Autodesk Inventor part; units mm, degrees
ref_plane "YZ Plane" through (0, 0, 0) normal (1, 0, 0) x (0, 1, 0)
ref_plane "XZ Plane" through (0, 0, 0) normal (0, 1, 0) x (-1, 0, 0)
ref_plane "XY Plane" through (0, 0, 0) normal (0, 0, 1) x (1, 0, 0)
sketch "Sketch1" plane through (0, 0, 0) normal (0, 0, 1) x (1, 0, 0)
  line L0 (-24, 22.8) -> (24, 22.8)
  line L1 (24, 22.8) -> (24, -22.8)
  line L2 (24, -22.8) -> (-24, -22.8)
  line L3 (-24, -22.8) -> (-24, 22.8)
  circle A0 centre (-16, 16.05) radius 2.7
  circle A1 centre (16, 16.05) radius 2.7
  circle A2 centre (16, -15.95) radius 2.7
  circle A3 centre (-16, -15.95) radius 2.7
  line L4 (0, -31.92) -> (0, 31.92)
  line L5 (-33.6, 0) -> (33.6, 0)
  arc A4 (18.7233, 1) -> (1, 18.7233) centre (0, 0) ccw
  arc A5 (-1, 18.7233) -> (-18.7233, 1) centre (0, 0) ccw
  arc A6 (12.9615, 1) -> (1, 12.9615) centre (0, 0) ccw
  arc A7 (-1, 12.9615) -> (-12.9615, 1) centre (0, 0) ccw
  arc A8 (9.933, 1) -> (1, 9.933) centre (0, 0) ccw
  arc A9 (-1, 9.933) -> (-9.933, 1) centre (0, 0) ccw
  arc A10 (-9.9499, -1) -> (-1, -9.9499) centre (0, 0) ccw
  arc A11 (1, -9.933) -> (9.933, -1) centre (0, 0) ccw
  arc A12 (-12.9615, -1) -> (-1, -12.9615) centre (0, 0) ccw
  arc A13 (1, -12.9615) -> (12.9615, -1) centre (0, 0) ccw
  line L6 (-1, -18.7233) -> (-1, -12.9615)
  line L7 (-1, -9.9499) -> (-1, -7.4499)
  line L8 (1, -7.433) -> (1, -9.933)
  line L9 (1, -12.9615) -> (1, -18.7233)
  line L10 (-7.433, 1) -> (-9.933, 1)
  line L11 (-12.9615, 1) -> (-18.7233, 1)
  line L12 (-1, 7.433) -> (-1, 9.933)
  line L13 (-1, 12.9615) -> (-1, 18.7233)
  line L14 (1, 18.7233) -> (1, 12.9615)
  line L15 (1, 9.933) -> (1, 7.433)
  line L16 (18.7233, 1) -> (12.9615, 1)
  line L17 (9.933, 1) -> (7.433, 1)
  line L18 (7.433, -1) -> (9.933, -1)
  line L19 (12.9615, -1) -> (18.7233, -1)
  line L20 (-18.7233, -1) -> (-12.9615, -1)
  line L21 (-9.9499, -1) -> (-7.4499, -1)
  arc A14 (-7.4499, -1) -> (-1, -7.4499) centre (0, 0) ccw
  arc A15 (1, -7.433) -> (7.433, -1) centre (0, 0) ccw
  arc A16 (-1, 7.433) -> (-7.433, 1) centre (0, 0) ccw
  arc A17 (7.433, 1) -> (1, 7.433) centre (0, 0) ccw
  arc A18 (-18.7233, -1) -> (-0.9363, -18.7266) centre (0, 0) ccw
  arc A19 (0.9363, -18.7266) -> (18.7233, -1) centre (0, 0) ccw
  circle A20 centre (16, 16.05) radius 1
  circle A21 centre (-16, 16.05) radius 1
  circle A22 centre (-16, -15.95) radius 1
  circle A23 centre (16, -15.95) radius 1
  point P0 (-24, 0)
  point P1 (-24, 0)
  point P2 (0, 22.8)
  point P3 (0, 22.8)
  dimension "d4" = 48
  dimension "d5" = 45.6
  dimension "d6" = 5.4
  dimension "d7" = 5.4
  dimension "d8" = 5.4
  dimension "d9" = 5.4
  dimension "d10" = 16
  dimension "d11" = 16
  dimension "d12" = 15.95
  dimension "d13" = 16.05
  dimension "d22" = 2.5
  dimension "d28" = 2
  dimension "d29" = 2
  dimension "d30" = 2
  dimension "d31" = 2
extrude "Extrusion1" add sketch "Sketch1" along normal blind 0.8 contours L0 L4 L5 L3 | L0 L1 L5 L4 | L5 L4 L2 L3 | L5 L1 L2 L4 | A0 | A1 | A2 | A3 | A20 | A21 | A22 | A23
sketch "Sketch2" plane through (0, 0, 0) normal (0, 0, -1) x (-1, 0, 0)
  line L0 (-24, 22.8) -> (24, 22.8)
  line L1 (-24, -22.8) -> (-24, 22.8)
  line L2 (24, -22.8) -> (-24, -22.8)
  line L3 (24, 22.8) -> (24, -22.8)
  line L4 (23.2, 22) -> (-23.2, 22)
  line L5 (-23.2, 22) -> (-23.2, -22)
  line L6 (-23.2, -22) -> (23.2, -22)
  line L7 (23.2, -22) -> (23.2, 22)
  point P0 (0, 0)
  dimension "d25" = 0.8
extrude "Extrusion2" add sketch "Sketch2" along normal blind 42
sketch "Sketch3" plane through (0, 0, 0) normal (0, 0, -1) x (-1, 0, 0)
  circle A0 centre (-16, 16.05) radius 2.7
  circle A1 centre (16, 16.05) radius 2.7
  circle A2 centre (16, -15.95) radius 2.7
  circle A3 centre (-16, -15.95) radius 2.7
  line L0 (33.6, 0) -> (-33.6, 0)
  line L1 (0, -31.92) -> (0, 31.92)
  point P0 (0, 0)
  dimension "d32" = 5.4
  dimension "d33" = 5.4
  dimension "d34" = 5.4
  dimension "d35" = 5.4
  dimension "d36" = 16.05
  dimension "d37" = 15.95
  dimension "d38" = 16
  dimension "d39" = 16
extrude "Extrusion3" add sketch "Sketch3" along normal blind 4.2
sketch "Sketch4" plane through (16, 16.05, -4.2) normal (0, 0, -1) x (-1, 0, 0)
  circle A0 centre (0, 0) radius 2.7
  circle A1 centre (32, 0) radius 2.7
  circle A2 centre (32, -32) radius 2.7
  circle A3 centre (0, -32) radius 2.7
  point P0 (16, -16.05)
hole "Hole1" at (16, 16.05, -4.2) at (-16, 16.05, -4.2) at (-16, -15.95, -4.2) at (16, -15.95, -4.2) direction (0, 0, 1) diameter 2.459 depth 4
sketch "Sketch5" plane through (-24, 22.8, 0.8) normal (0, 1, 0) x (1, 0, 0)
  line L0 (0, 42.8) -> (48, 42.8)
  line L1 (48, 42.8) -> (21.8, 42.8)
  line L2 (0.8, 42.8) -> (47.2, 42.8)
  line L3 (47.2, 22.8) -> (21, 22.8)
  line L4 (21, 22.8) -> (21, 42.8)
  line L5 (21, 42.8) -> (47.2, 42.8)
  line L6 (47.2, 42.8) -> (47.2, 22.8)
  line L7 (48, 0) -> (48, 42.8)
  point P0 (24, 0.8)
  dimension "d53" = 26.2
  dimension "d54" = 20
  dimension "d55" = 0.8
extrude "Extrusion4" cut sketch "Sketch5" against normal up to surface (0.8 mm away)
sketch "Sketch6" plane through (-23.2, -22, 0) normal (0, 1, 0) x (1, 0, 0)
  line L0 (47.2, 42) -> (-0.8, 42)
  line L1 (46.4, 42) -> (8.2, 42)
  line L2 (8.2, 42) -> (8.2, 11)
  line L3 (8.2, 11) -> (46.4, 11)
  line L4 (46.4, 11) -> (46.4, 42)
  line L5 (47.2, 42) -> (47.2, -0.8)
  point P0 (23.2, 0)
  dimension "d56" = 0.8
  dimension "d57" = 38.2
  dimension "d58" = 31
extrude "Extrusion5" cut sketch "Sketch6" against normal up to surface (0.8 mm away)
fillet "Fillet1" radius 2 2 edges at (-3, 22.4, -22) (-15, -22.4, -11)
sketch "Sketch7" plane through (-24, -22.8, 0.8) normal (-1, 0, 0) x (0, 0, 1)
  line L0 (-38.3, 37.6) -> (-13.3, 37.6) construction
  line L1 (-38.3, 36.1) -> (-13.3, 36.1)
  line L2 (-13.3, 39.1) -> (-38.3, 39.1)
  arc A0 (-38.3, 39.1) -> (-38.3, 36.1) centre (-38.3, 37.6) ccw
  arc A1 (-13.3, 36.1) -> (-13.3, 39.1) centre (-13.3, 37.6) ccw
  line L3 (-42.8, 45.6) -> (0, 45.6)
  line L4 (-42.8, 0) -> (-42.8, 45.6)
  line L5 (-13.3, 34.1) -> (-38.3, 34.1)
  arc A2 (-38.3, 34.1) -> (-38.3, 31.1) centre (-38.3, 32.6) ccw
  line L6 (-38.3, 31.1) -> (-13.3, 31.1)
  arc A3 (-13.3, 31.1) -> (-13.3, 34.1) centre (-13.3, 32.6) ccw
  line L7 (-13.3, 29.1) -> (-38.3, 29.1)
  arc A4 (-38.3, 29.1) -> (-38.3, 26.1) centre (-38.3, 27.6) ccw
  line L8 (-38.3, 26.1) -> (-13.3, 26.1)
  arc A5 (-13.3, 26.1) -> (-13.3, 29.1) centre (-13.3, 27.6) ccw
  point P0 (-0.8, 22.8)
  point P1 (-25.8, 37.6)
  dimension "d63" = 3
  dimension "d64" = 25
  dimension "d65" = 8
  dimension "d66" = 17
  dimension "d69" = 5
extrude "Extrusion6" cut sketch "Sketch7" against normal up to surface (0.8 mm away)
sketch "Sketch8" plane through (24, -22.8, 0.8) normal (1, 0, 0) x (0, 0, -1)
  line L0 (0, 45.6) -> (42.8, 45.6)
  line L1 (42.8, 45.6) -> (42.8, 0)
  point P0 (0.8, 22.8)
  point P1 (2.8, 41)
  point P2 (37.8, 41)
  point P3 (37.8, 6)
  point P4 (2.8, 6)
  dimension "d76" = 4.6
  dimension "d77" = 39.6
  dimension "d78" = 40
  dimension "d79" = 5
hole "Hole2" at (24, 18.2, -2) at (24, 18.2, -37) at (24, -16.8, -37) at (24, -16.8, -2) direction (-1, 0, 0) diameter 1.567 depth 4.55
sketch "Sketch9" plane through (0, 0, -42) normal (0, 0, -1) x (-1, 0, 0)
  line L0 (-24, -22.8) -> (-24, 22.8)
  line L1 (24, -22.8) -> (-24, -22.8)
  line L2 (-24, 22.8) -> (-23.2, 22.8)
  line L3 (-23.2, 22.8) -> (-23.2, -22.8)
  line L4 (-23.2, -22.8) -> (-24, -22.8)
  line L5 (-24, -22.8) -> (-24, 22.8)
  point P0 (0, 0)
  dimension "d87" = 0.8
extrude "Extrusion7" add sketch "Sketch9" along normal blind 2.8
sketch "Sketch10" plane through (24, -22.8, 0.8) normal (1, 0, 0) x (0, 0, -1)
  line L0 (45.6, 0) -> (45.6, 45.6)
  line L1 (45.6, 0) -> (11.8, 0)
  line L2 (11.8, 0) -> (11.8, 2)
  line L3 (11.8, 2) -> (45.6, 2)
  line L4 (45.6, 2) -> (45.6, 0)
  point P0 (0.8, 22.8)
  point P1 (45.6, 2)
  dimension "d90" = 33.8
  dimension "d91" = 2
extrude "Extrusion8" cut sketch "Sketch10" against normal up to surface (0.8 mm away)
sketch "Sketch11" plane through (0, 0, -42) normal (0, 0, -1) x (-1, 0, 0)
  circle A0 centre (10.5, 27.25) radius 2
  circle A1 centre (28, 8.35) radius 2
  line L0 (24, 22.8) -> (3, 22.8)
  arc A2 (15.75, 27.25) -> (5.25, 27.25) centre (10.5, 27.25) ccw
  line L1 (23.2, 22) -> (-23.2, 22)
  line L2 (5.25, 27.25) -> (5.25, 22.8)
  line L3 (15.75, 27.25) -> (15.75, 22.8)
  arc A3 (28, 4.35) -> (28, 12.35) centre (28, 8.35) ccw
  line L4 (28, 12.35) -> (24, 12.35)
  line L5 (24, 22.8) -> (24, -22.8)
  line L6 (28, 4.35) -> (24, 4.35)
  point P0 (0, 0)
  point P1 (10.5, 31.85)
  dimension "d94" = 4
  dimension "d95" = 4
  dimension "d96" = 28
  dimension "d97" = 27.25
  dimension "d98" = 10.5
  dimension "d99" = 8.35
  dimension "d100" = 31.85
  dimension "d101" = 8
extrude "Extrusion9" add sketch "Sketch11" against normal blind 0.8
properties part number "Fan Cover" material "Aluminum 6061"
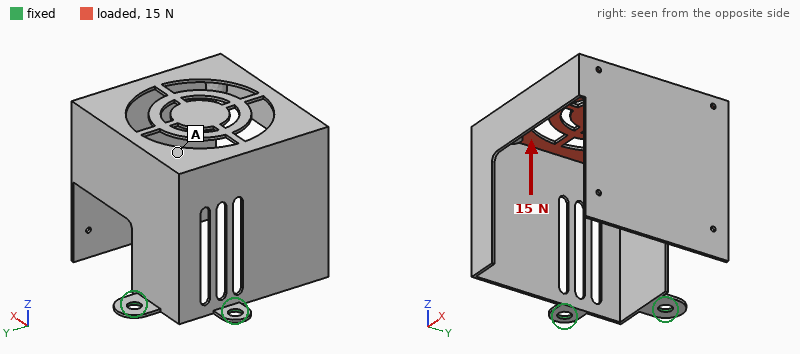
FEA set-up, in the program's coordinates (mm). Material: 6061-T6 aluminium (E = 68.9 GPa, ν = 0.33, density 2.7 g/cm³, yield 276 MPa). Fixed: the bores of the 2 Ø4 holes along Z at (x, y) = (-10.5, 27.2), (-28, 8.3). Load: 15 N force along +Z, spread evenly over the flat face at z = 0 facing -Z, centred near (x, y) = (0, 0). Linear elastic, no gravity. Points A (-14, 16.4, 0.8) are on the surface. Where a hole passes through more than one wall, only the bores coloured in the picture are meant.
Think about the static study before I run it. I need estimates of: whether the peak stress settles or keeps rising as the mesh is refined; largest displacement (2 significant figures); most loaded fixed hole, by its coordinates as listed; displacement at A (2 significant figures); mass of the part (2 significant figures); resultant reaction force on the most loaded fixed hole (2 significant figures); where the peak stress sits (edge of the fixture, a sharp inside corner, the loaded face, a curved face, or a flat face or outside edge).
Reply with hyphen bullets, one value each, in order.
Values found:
- keeps rising
- 1.0 mm
- (-28, 8.3)
- 0.44 mm
- 17 g
- 9.4 N
- edge of the fixture
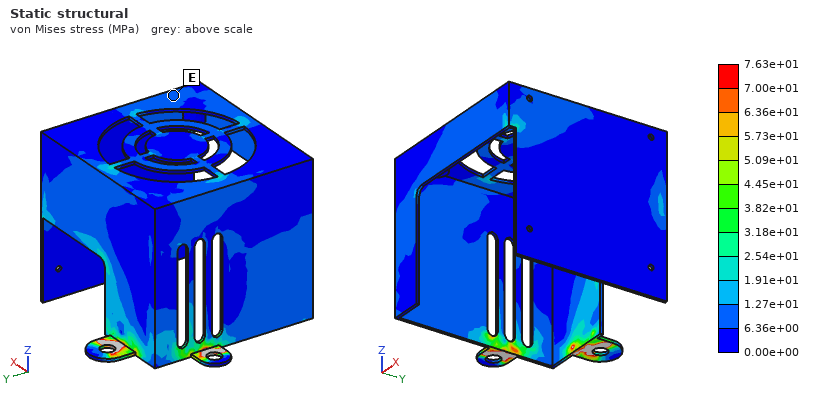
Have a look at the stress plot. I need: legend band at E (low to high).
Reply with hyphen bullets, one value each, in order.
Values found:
- 6.36e+00 to 1.27e+01 MPa
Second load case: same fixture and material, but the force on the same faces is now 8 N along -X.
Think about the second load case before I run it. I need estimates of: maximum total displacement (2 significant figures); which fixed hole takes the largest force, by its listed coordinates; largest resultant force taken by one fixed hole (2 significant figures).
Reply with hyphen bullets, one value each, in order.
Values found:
- 1.0 mm
- (-28, 8.3)
- 10 N
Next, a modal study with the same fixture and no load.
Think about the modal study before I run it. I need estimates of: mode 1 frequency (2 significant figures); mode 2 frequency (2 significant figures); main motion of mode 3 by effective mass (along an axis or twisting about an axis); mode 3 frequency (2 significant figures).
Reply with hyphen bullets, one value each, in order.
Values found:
- 110 Hz
- 170 Hz
- along X
- 320 Hz
